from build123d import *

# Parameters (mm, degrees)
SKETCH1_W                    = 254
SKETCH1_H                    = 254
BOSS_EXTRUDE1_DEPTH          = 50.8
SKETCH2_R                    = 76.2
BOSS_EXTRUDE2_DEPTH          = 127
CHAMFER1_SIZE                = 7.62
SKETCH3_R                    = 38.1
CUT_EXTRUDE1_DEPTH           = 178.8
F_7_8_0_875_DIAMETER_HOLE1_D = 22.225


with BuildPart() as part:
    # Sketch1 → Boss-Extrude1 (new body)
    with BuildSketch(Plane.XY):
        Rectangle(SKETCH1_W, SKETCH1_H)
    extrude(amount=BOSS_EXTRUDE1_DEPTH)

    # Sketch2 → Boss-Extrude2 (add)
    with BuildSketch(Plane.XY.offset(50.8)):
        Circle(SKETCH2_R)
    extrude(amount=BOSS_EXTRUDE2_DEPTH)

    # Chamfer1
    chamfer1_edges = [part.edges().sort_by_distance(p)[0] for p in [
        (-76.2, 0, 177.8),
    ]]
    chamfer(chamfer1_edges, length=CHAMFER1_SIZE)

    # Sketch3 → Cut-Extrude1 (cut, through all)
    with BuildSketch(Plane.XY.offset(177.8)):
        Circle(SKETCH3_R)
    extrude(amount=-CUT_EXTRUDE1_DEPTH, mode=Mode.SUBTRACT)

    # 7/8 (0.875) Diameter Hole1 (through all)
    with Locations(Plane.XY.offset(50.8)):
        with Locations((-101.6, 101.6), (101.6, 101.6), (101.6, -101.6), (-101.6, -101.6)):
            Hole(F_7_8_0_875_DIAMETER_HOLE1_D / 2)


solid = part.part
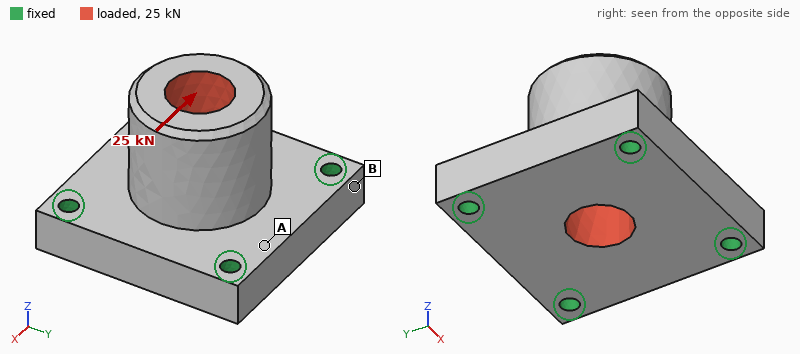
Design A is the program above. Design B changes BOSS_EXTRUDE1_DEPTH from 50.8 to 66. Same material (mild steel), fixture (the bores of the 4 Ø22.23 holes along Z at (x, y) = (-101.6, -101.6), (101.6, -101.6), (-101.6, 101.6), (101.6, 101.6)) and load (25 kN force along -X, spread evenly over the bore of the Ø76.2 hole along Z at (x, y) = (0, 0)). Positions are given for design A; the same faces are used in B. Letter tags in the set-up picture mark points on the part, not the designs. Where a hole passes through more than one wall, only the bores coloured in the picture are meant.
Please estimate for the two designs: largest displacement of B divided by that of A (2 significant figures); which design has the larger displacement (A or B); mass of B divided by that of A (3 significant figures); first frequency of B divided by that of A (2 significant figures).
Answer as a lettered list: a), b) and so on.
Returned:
a) 0.62
b) A
c) 1.14
d) 1.3
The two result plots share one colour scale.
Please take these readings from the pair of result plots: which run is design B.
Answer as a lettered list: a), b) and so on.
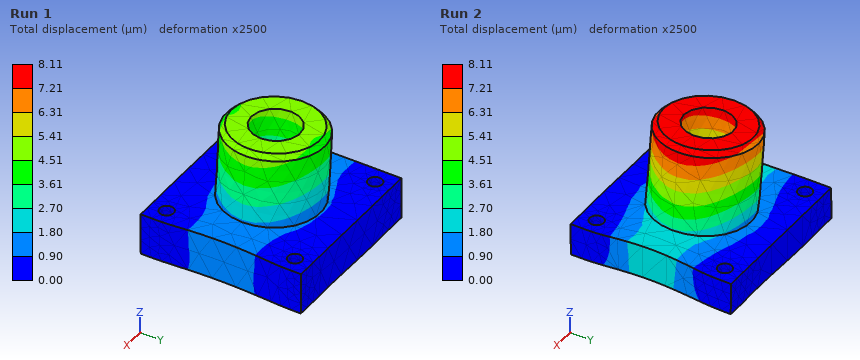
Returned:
a) Run 1
